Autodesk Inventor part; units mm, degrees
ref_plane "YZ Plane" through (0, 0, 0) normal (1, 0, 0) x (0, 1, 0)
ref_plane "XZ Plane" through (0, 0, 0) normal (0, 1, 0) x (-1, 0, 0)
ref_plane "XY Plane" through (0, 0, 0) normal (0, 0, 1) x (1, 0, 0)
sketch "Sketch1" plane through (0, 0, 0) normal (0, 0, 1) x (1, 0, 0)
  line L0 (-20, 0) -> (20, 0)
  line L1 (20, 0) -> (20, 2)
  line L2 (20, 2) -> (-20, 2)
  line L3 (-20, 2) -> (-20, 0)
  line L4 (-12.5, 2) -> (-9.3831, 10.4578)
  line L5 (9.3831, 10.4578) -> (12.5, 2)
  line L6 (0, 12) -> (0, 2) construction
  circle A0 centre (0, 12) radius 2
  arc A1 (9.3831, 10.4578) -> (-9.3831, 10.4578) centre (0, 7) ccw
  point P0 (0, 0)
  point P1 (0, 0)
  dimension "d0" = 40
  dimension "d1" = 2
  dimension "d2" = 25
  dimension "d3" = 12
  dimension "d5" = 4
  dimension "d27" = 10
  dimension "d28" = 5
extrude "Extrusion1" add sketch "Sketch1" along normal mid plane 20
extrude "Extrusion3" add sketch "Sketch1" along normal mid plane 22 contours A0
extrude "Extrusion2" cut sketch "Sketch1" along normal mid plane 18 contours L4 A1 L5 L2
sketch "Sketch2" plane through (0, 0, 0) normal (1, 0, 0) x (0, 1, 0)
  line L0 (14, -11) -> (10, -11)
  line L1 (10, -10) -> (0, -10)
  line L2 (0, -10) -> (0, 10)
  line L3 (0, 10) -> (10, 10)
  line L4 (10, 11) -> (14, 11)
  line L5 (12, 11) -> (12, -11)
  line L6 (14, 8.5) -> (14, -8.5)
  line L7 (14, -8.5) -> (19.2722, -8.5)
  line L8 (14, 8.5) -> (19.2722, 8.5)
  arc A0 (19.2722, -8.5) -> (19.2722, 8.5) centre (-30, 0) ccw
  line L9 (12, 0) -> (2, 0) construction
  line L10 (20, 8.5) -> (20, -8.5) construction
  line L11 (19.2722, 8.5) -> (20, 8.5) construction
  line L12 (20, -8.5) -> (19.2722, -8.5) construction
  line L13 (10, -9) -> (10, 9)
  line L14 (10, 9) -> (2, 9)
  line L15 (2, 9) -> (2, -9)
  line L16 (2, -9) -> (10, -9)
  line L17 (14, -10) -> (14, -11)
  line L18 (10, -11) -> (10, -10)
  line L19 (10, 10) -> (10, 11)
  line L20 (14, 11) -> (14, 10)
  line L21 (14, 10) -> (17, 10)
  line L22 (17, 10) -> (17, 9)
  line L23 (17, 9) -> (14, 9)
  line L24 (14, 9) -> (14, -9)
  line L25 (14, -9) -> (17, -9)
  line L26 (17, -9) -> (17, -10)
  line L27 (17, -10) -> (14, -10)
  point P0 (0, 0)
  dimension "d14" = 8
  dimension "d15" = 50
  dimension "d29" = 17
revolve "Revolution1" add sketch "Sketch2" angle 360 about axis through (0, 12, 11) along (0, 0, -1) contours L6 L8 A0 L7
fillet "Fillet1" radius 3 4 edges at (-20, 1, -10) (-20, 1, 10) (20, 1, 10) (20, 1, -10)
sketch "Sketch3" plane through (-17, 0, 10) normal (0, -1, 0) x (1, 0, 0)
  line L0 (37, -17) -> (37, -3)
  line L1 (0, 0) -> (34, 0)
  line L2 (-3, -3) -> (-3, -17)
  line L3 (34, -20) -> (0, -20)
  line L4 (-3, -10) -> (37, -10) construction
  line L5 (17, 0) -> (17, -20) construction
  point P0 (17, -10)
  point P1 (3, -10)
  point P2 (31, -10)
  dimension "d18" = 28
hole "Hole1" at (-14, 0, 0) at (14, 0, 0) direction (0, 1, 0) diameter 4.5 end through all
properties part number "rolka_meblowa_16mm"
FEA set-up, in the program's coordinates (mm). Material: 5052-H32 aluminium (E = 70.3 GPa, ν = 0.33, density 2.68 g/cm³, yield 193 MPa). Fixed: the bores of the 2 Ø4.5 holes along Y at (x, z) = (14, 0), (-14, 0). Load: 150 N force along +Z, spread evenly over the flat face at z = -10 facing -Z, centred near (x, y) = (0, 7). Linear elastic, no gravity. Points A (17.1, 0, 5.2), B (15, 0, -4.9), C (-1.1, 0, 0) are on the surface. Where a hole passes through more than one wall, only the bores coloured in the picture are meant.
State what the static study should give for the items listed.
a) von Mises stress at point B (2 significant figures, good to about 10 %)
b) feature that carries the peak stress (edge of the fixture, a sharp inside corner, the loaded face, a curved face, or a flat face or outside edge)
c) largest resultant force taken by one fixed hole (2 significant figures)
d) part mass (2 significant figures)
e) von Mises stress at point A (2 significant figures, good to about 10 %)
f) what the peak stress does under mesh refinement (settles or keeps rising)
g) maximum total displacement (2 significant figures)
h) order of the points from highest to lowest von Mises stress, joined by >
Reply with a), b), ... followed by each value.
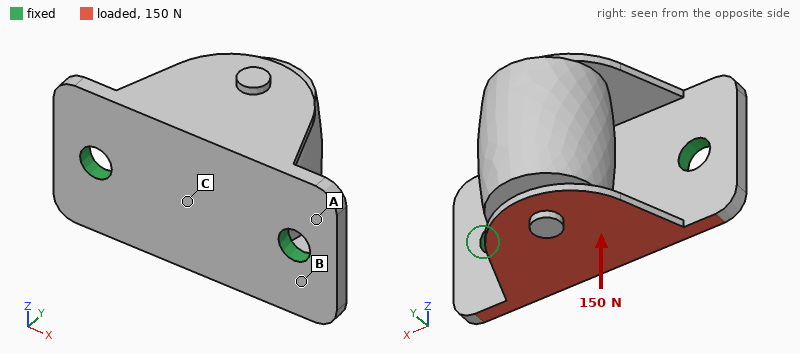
a) 17 MPa
b) a sharp inside corner
c) 75 N
d) 14 g
e) 11 MPa
f) keeps rising
g) 60 µm
h) B > A > C
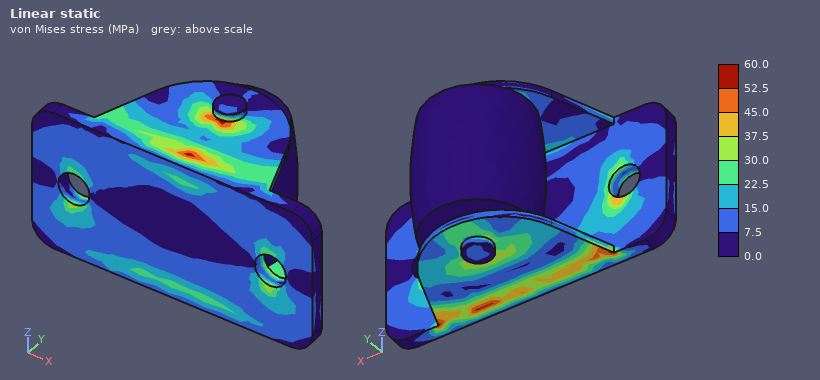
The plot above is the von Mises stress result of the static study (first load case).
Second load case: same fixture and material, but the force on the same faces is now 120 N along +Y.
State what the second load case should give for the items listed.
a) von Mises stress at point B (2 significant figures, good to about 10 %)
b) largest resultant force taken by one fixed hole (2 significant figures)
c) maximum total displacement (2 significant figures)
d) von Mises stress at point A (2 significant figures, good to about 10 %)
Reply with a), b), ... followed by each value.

a) 31 MPa
b) 61 N
c) 33 µm
d) 5.9 MPa
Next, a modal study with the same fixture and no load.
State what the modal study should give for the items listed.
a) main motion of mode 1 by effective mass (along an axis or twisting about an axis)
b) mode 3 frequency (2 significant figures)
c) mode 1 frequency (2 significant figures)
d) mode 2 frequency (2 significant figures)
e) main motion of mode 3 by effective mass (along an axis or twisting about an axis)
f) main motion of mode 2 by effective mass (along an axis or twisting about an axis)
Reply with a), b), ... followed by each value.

a) along Z
b) 5500 Hz
c) 2000 Hz
d) 5300 Hz
e) along Y
f) along X
